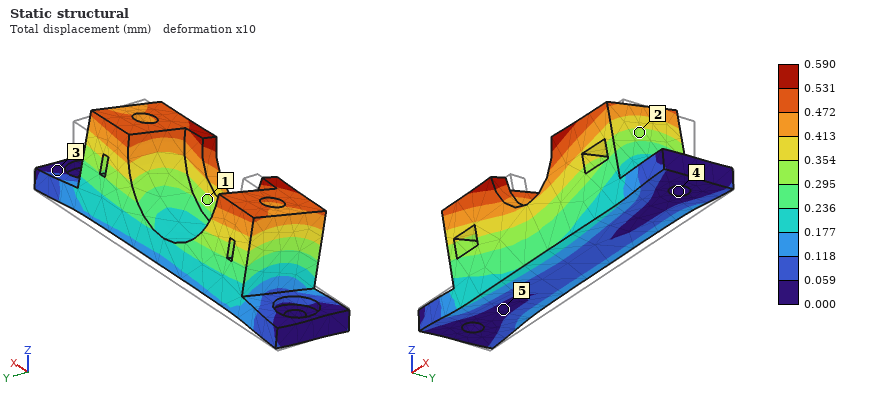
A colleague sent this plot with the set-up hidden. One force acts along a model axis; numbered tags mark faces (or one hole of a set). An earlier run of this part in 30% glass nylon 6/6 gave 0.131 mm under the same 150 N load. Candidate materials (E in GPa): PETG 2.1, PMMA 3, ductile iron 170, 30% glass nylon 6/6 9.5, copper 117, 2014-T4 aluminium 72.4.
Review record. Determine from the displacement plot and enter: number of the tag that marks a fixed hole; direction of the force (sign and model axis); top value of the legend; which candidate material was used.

4
-Y
0.590 mm
PETG
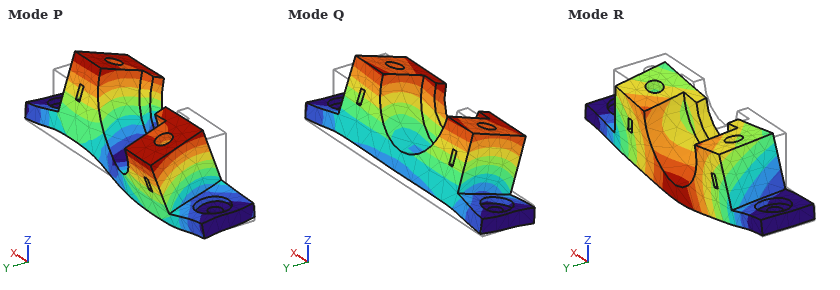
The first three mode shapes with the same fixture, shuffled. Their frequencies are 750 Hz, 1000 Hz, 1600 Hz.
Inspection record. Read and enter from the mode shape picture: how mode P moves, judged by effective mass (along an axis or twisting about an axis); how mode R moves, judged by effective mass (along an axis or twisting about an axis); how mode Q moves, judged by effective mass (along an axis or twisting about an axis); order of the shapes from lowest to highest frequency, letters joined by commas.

twisting about Z
along Z
along Y
Q, R, P
